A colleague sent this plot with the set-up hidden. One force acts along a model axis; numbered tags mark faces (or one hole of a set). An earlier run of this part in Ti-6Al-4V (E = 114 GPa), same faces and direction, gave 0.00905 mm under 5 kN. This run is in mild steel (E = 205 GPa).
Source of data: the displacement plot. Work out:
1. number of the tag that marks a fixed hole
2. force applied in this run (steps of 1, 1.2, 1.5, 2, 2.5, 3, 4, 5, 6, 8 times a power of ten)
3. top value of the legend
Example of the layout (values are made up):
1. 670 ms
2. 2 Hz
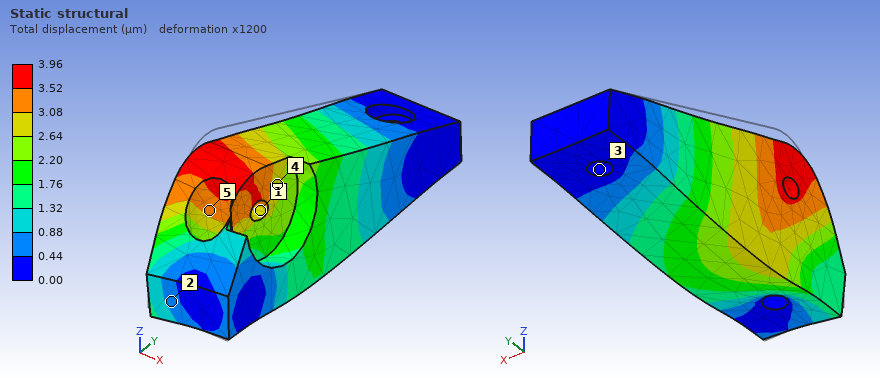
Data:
1. 3
2. 4 kN
3. 3.96 µm
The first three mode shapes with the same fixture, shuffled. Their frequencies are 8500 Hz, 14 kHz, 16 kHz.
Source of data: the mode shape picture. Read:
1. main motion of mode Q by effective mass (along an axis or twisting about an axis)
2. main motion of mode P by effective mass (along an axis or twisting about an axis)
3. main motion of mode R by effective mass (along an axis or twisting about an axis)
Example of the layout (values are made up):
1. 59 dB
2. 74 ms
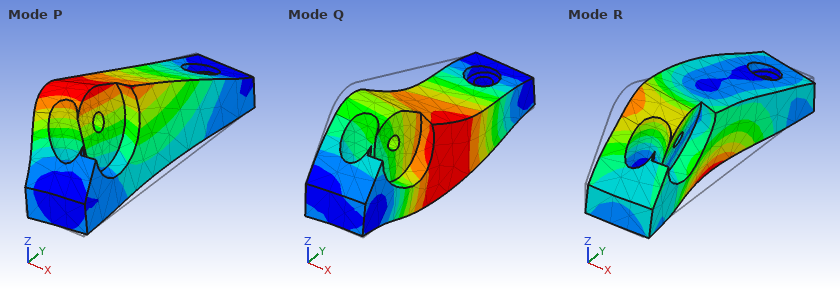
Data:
1. along Z
2. along X
3. along X
